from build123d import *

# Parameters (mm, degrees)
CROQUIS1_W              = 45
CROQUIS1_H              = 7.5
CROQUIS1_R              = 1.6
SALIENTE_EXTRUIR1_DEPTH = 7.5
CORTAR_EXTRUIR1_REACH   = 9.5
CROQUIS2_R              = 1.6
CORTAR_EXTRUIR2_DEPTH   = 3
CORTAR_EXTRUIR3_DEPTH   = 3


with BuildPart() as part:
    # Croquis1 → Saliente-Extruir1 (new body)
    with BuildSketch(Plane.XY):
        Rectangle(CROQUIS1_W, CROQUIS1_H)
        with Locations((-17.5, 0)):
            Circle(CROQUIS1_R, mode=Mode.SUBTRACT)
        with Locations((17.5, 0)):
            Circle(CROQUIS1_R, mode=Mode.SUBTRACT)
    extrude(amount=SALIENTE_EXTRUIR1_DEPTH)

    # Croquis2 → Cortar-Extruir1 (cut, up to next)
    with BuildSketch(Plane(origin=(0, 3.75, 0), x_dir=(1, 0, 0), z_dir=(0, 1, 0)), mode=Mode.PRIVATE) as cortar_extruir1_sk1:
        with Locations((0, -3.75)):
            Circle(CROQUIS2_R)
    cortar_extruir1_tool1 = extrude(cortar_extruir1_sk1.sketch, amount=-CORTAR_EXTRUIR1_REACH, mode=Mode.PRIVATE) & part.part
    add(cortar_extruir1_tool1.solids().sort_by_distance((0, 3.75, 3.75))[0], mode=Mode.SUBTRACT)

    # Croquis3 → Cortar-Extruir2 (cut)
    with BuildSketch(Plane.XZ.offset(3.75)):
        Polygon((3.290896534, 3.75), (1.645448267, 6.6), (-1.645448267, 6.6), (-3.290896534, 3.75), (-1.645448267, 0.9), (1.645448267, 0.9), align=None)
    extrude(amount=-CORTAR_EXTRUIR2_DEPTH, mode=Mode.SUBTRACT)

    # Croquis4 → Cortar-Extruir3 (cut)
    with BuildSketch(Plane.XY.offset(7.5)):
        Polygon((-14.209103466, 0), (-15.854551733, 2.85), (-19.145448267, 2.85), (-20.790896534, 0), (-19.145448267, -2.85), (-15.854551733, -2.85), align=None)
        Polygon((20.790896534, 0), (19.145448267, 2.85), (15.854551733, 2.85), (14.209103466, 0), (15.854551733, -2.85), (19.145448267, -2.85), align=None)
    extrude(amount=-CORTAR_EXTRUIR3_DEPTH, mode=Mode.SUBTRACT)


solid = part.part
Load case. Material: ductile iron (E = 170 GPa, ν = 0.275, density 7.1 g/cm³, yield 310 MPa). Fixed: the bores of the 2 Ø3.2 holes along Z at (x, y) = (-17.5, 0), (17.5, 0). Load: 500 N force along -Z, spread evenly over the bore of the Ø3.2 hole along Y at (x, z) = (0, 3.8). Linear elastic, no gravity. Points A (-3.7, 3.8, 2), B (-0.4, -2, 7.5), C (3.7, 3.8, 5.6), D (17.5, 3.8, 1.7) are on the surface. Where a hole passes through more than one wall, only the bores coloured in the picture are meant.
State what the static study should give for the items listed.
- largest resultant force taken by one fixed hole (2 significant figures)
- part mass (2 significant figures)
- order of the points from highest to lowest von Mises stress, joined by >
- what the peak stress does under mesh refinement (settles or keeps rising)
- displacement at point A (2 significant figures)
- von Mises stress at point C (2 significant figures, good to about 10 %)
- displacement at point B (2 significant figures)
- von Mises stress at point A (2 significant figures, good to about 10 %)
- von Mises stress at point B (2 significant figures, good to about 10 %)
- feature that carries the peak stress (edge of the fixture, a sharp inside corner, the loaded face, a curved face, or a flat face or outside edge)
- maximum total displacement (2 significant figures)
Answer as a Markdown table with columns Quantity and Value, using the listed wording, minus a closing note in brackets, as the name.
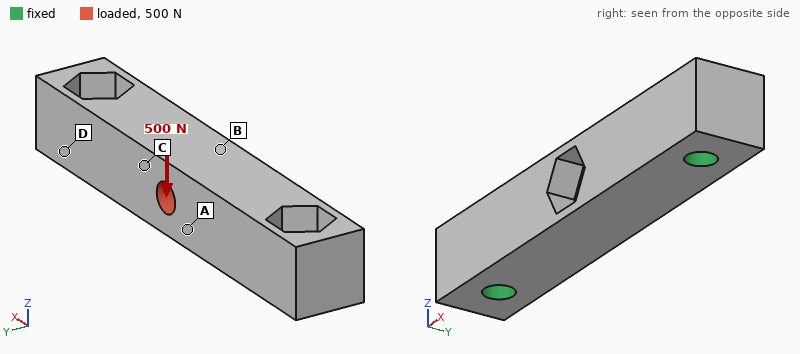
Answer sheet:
| Quantity | Value |
|---|---|
| largest resultant force taken by one fixed hole | 290 N |
| part mass | 15 g |
| order of the points from highest to lowest von Mises stress, joined by > | B > C > A > D |
| what the peak stress does under mesh refinement | keeps rising |
| displacement at point A | 5.3 µm |
| von Mises stress at point C | 23 MPa |
| displacement at point B | 4.3 µm |
| von Mises stress at point A | 17 MPa |
| von Mises stress at point B | 45 MPa |
| feature that carries the peak stress | edge of the fixture |
| maximum total displacement | 6.2 µm |
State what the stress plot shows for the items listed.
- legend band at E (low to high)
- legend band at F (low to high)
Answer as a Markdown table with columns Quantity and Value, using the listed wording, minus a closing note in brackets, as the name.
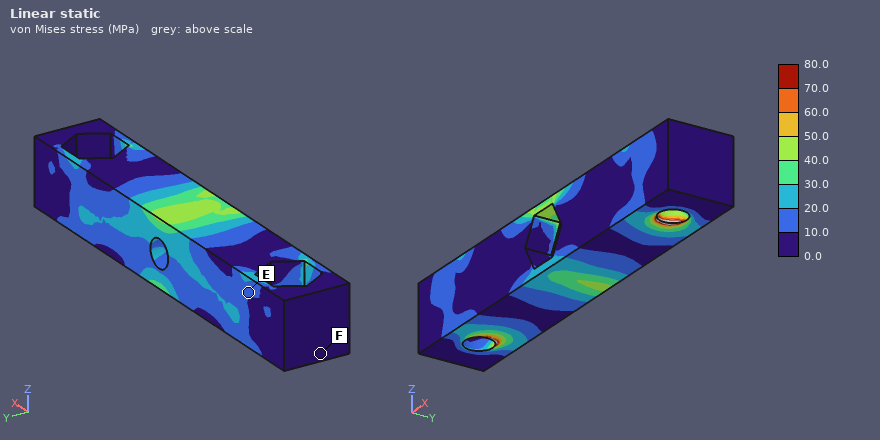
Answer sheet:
| Quantity | Value |
|---|---|
| legend band at E | 10.0 to 20.0 MPa |
| legend band at F | 0.0 to 10.0 MPa |
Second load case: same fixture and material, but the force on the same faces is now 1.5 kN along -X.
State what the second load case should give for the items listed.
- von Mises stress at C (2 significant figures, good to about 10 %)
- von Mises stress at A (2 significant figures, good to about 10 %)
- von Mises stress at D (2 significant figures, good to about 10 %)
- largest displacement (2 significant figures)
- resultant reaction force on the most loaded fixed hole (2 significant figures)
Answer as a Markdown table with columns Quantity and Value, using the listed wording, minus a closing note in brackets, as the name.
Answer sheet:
| Quantity | Value |
|---|---|
| von Mises stress at C | 23 MPa |
| von Mises stress at A | 26 MPa |
| von Mises stress at D | 6.5 MPa |
| largest displacement | 2.1 µm |
| resultant reaction force on the most loaded fixed hole | 760 N |
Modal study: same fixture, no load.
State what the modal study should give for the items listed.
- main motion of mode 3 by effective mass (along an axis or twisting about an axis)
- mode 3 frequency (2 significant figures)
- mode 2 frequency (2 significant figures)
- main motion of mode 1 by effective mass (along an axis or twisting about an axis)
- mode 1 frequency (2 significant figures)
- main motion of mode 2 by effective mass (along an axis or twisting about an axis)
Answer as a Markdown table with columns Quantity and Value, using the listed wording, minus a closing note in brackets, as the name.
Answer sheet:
| Quantity | Value |
|---|---|
| main motion of mode 3 by effective mass | twisting about X |
| mode 3 frequency | 35 kHz |
| mode 2 frequency | 22 kHz |
| main motion of mode 1 by effective mass | along Y |
| mode 1 frequency | 20 kHz |
| main motion of mode 2 by effective mass | along Z |
